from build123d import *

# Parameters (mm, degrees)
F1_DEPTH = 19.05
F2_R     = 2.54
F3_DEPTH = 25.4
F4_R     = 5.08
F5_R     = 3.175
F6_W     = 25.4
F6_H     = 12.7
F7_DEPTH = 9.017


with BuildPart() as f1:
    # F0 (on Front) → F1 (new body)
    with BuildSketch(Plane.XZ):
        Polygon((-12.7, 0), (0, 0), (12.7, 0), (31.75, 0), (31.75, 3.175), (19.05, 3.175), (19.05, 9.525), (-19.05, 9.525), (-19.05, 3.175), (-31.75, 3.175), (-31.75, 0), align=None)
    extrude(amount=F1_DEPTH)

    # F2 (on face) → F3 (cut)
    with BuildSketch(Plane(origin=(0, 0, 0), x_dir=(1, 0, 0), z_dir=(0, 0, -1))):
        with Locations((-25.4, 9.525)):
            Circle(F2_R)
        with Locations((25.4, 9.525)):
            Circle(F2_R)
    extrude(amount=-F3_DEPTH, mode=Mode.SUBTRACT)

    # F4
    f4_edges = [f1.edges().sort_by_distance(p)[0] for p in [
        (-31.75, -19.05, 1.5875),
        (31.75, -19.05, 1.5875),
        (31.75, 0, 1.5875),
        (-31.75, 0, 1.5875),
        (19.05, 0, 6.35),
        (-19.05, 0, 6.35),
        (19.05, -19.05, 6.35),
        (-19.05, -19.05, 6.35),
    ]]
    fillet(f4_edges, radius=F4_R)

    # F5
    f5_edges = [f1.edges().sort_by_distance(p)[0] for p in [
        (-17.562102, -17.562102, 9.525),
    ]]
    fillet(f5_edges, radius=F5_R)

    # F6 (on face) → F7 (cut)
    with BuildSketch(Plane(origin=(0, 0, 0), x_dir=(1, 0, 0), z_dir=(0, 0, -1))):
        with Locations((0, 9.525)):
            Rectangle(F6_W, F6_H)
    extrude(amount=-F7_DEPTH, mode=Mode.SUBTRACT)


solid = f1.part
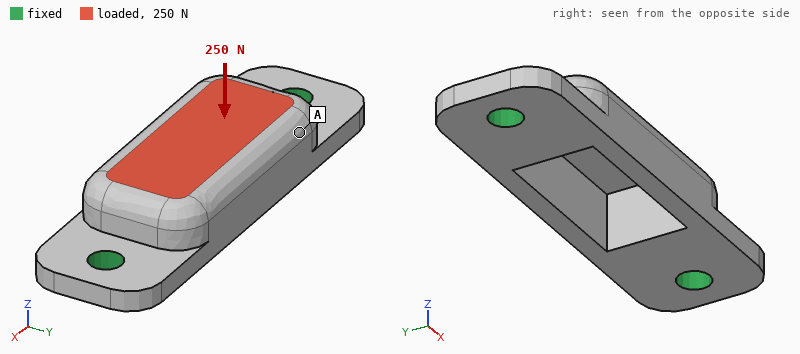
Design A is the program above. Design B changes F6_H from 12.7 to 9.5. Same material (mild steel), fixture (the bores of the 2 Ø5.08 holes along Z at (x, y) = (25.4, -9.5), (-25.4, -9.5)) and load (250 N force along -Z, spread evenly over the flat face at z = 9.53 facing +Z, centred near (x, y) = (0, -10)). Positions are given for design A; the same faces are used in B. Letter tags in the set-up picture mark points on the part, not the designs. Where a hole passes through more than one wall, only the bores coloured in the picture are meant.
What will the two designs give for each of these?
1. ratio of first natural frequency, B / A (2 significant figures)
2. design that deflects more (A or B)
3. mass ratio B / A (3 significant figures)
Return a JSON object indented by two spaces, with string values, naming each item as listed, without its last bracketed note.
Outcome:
{
  "ratio of first natural frequency, B / A": "0.93",
  "design that deflects more": "A",
  "mass ratio B / A": "1.15"
}
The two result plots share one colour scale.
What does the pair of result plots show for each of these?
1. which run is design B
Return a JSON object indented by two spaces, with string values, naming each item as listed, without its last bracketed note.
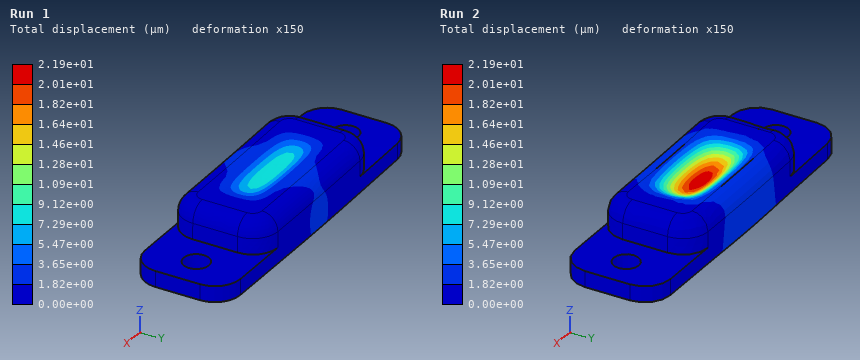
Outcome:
{
  "which run is design B": "Run 1"
}
